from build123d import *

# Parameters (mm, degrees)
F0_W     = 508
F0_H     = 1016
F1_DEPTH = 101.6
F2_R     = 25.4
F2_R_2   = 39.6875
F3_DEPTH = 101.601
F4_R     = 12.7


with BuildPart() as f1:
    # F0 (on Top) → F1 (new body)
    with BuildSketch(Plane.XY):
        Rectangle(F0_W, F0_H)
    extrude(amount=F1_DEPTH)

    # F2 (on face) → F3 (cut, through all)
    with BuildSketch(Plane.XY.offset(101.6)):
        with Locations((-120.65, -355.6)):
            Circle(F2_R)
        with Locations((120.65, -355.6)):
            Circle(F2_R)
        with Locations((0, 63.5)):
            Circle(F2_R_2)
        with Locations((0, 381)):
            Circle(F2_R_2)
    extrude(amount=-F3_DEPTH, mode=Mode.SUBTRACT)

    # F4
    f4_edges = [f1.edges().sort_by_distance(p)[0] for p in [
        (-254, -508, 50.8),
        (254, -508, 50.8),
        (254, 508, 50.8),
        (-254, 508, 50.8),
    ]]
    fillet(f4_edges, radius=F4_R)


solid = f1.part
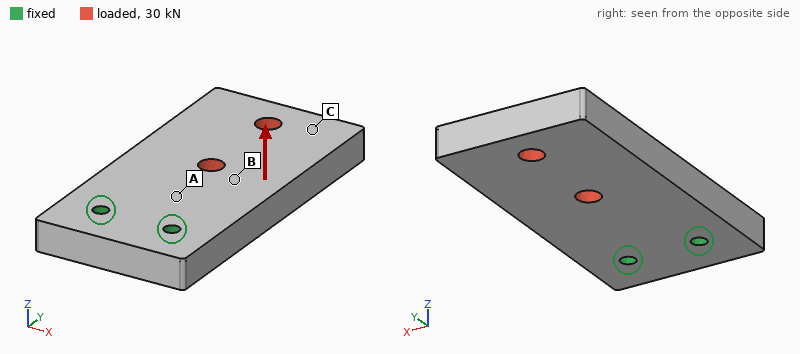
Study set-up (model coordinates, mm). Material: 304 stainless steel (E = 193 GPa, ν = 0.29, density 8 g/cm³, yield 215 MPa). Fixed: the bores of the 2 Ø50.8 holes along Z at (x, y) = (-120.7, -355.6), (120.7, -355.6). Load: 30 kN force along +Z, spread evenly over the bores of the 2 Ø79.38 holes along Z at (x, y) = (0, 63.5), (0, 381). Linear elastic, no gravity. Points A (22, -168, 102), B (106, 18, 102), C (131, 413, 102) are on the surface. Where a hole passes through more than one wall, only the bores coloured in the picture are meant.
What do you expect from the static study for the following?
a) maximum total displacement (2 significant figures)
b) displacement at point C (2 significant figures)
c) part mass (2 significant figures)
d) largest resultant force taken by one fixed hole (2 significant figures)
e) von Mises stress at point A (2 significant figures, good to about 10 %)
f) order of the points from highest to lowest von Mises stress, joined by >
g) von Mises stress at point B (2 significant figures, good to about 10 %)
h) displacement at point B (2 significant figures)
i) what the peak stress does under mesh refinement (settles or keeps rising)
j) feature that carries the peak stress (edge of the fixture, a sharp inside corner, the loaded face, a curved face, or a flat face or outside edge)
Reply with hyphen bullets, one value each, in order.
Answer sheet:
- 0.44 mm
- 0.37 mm
- 410 kg
- 15 kN
- 12 MPa
- A > B > C
- 7.7 MPa
- 0.13 mm
- keeps rising
- edge of the fixture
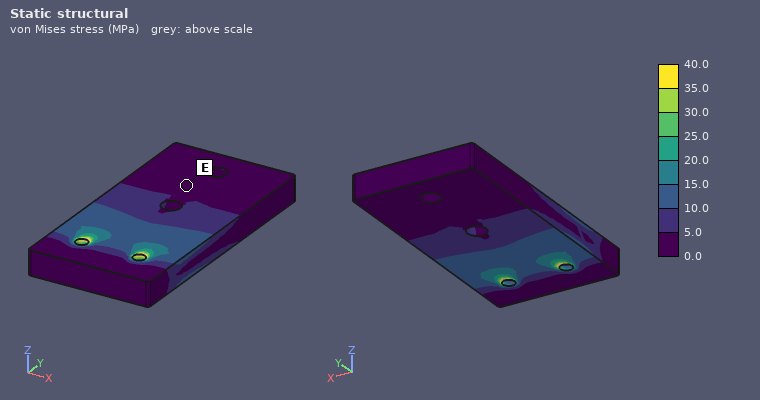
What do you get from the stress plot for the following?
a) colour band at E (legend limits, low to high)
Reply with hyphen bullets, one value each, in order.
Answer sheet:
- 0.0 to 5.0 MPa
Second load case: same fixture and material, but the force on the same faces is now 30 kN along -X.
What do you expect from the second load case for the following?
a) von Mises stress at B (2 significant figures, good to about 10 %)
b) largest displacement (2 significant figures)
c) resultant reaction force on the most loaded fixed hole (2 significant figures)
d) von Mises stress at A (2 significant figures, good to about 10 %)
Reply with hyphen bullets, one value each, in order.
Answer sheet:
- 1.4 MPa
- 31 µm
- 65 kN
- 2.0 MPa
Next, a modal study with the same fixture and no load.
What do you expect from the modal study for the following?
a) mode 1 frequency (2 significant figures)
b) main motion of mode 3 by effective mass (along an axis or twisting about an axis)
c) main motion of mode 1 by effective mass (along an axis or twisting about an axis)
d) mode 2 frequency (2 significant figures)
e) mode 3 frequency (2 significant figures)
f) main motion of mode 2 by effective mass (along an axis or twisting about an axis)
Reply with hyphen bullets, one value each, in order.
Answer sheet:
- 110 Hz
- along X
- along Z
- 360 Hz
- 380 Hz
- twisting about Y
